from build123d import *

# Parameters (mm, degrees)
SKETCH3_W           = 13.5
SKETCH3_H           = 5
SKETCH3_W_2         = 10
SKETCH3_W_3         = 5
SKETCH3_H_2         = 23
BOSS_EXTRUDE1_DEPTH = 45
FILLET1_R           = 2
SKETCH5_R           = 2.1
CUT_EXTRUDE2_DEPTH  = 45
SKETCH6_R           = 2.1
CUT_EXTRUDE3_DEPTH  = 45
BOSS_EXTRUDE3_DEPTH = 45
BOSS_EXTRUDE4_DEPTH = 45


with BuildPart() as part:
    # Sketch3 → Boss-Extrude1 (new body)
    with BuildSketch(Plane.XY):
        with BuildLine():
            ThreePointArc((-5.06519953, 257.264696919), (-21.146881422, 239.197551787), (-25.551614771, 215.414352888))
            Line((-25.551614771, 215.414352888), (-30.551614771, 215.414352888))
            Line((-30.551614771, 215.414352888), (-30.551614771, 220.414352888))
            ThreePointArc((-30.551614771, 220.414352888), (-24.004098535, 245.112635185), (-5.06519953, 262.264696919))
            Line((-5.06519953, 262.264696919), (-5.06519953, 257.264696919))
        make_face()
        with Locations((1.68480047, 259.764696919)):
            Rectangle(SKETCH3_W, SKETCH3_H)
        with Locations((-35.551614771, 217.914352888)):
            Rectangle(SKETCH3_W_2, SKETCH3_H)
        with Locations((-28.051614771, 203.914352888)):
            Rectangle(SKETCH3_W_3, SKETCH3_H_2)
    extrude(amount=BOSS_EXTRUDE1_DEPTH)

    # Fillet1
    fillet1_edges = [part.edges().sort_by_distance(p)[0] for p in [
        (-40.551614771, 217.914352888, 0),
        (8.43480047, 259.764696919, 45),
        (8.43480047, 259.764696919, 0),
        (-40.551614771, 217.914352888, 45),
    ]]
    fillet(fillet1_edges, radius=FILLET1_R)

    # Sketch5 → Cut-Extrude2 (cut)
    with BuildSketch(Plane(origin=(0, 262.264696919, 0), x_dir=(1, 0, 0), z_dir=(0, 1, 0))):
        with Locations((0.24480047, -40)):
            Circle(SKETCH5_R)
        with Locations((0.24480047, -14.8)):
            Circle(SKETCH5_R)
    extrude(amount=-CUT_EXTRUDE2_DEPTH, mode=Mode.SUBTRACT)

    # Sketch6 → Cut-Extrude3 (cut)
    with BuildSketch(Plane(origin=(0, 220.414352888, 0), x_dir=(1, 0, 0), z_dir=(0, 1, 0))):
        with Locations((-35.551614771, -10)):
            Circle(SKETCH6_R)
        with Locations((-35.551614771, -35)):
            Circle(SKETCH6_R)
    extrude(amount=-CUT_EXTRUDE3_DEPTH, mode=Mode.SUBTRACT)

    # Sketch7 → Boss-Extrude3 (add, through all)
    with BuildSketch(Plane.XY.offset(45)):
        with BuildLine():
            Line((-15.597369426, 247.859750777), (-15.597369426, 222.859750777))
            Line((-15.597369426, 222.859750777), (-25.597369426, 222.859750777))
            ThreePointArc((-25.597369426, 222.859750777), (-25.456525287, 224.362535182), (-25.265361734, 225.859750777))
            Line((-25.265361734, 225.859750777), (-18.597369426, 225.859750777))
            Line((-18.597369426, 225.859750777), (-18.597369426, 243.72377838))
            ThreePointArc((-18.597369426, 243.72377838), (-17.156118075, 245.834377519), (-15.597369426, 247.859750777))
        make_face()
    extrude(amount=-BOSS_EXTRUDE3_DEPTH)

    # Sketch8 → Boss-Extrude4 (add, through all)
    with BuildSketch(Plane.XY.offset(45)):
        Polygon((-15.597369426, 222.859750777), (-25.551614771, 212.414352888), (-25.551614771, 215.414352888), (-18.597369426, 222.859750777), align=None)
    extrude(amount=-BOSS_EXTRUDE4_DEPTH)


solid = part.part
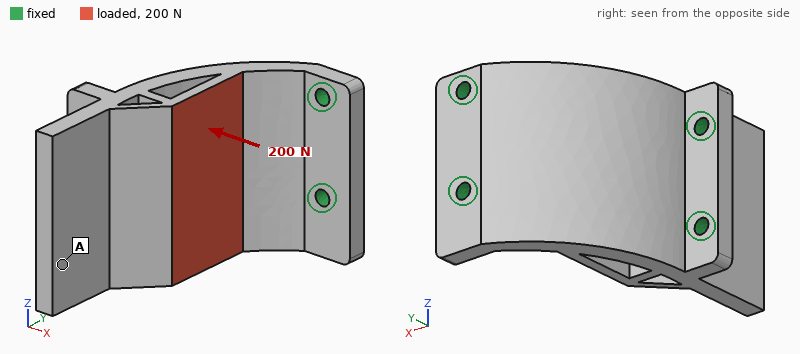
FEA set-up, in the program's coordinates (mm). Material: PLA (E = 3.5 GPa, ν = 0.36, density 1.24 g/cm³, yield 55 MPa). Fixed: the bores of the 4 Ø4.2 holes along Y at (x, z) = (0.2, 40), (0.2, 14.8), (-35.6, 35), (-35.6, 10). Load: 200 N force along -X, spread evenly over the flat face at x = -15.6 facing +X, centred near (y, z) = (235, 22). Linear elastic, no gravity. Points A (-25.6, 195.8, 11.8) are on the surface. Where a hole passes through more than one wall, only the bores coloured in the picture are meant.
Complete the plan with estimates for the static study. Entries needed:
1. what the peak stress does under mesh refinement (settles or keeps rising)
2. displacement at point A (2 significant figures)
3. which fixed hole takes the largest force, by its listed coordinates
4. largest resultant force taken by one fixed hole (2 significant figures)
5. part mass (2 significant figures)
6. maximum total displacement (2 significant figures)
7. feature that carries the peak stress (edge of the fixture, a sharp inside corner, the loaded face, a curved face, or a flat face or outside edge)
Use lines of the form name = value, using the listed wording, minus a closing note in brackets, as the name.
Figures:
what the peak stress does under mesh refinement = keeps rising
displacement at point A = 20 µm
which fixed hole takes the largest force, by its listed coordinates = (0.2, 14.8)
largest resultant force taken by one fixed hole = 84 N
part mass = 34 g
maximum total displacement = 42 µm
feature that carries the peak stress = edge of the fixture
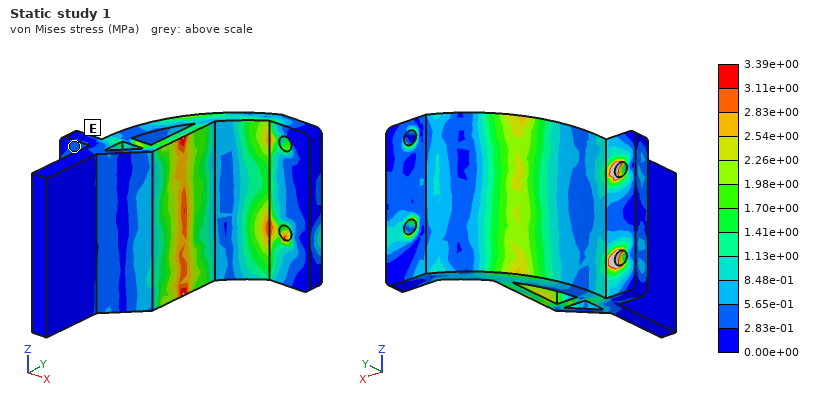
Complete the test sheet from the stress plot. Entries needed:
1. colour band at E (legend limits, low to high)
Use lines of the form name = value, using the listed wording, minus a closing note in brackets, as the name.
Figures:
colour band at E = 2.83e-01 to 5.65e-01 MPa
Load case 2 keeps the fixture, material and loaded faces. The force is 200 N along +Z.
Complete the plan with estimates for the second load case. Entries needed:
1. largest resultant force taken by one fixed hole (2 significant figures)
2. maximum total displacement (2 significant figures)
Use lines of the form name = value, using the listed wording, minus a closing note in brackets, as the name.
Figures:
largest resultant force taken by one fixed hole = 84 N
maximum total displacement = 20 µm
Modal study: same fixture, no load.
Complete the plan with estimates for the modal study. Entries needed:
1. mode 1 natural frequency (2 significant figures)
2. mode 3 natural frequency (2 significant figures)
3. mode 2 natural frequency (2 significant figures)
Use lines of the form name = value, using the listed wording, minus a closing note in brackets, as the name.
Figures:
mode 1 natural frequency = 2100 Hz
mode 3 natural frequency = 3400 Hz
mode 2 natural frequency = 3200 Hz
